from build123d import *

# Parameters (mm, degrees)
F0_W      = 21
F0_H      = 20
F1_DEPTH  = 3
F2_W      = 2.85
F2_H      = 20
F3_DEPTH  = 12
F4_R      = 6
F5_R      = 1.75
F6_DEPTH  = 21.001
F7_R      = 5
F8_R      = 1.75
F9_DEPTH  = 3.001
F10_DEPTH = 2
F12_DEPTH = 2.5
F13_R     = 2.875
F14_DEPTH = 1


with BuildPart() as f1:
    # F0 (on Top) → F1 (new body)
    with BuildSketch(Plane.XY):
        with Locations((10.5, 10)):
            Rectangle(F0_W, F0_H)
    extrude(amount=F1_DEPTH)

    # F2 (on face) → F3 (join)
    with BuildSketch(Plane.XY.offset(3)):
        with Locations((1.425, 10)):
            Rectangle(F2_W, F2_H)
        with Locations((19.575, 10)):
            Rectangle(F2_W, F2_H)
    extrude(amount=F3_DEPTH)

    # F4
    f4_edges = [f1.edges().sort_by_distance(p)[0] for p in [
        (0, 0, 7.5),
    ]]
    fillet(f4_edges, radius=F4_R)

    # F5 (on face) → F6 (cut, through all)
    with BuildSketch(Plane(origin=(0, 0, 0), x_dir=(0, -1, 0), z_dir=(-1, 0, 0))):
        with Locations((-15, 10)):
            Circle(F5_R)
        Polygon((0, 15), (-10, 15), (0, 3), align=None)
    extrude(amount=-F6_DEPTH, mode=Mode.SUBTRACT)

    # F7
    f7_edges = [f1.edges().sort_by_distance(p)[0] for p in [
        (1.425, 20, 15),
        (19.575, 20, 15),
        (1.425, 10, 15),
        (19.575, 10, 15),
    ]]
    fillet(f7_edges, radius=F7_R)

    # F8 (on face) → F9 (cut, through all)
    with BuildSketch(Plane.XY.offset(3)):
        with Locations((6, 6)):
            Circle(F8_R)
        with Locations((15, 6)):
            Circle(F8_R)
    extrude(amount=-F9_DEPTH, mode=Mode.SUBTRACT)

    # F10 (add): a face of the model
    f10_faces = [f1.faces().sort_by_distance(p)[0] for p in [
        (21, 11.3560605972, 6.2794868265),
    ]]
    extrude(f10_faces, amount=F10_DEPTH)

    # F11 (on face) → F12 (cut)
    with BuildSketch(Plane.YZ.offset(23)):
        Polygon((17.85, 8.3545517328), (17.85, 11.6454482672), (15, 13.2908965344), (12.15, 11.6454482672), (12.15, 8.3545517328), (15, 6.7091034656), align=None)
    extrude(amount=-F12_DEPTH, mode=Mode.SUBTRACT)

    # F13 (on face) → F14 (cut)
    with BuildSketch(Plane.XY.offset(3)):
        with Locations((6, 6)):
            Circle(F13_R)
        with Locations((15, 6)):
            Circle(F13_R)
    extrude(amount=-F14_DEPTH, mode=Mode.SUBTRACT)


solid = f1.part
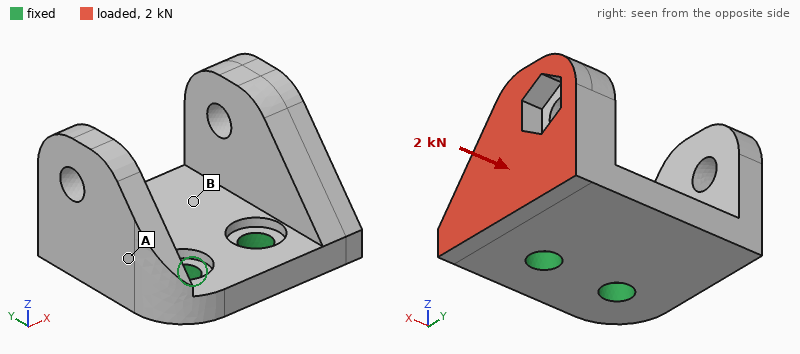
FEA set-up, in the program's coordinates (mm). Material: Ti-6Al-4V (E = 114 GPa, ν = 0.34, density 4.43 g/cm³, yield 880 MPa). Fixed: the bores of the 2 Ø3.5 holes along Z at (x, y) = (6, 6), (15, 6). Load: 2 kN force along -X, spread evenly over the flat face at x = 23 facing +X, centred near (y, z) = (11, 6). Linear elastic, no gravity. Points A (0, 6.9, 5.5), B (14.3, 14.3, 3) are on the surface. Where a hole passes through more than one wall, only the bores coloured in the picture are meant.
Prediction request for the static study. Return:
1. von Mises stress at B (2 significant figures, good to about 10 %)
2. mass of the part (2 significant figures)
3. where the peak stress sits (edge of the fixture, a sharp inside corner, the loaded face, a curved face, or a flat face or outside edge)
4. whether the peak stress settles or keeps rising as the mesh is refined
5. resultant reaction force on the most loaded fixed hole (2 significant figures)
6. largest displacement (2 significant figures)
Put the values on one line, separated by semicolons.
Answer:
240 MPa; 11 g; edge of the fixture; keeps rising; 1.4 kN; 0.21 mm
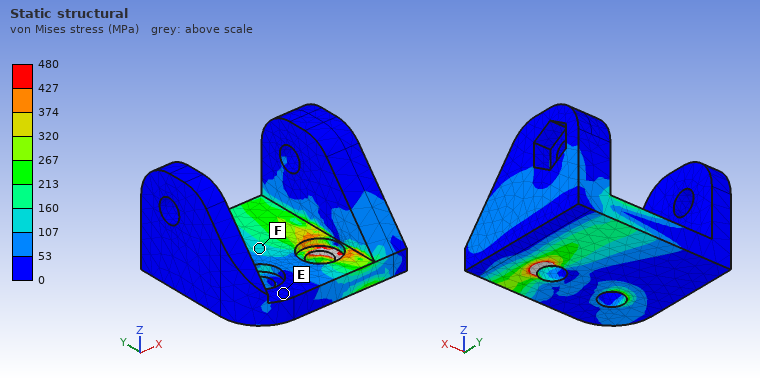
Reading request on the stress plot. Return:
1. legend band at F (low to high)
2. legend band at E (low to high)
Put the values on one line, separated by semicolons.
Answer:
107 to 160 MPa; 0 to 53 MPa
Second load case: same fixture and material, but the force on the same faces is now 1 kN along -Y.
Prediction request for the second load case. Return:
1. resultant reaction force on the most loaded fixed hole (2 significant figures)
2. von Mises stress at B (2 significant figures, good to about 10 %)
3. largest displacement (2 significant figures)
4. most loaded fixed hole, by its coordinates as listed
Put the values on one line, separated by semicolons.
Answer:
1.5 kN; 36 MPa; 74 µm; (15, 6)
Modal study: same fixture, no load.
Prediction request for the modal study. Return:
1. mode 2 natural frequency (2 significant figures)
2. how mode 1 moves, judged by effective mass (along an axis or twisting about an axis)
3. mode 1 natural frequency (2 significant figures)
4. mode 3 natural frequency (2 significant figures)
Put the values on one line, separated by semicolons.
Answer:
8000 Hz; along Z; 6900 Hz; 9700 Hz
